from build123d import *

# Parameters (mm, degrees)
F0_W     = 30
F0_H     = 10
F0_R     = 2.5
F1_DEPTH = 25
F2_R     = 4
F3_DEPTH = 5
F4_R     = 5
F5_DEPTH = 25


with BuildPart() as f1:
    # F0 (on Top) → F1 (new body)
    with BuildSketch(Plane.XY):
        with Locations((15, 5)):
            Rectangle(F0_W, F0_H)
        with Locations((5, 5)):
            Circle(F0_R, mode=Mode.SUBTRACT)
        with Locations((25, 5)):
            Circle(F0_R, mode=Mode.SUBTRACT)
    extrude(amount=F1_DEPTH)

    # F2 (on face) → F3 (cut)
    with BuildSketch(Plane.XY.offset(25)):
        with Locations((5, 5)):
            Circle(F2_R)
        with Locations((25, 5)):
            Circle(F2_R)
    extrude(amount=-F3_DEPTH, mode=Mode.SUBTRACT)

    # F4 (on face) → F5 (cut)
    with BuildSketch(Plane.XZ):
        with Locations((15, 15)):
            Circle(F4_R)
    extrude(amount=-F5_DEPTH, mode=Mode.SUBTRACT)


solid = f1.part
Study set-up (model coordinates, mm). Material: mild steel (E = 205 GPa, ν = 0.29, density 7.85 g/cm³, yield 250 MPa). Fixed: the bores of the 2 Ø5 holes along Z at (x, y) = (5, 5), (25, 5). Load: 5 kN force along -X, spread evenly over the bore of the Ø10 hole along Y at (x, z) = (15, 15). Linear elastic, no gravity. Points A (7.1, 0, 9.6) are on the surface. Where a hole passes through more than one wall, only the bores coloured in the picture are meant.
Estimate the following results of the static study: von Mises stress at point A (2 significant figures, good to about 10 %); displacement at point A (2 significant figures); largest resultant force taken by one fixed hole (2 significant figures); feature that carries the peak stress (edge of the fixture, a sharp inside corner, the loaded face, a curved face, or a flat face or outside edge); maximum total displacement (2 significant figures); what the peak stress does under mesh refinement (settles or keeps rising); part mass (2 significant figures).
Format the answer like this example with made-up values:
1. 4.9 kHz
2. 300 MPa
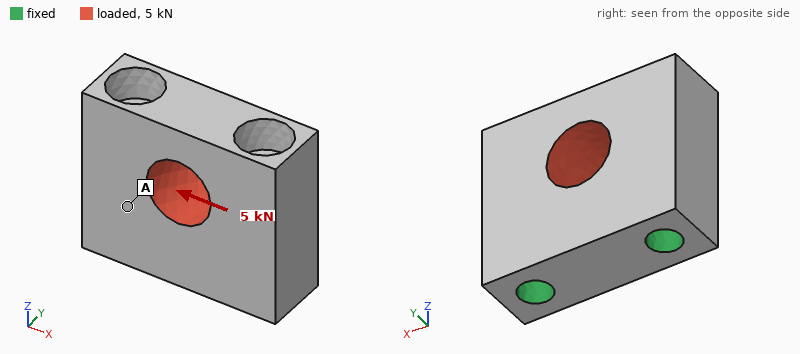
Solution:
1. 8.2 MPa
2. 0.18 µm
3. 2.5 kN
4. edge of the fixture
5. 1.1 µm
6. keeps rising
7. 43 g
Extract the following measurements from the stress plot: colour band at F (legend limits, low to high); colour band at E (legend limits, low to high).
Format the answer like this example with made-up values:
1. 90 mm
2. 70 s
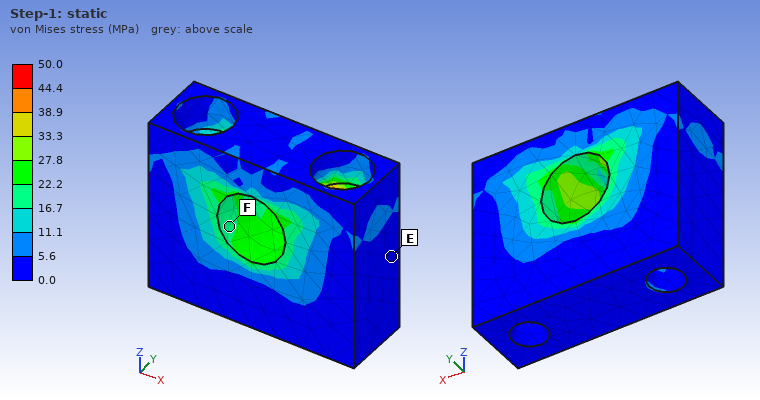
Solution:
1. 16.7 to 22.2 MPa
2. 0.0 to 5.6 MPa
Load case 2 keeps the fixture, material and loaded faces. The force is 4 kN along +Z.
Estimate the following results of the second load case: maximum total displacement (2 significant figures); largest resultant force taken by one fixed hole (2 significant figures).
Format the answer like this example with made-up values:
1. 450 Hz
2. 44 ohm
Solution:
1. 1.5 µm
2. 2.0 kN
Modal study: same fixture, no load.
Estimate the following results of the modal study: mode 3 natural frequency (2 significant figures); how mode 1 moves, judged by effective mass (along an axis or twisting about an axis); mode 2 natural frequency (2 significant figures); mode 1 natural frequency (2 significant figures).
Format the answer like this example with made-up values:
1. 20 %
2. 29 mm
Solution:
1. 74 kHz
2. along Y
3. 73 kHz
4. 45 kHz
